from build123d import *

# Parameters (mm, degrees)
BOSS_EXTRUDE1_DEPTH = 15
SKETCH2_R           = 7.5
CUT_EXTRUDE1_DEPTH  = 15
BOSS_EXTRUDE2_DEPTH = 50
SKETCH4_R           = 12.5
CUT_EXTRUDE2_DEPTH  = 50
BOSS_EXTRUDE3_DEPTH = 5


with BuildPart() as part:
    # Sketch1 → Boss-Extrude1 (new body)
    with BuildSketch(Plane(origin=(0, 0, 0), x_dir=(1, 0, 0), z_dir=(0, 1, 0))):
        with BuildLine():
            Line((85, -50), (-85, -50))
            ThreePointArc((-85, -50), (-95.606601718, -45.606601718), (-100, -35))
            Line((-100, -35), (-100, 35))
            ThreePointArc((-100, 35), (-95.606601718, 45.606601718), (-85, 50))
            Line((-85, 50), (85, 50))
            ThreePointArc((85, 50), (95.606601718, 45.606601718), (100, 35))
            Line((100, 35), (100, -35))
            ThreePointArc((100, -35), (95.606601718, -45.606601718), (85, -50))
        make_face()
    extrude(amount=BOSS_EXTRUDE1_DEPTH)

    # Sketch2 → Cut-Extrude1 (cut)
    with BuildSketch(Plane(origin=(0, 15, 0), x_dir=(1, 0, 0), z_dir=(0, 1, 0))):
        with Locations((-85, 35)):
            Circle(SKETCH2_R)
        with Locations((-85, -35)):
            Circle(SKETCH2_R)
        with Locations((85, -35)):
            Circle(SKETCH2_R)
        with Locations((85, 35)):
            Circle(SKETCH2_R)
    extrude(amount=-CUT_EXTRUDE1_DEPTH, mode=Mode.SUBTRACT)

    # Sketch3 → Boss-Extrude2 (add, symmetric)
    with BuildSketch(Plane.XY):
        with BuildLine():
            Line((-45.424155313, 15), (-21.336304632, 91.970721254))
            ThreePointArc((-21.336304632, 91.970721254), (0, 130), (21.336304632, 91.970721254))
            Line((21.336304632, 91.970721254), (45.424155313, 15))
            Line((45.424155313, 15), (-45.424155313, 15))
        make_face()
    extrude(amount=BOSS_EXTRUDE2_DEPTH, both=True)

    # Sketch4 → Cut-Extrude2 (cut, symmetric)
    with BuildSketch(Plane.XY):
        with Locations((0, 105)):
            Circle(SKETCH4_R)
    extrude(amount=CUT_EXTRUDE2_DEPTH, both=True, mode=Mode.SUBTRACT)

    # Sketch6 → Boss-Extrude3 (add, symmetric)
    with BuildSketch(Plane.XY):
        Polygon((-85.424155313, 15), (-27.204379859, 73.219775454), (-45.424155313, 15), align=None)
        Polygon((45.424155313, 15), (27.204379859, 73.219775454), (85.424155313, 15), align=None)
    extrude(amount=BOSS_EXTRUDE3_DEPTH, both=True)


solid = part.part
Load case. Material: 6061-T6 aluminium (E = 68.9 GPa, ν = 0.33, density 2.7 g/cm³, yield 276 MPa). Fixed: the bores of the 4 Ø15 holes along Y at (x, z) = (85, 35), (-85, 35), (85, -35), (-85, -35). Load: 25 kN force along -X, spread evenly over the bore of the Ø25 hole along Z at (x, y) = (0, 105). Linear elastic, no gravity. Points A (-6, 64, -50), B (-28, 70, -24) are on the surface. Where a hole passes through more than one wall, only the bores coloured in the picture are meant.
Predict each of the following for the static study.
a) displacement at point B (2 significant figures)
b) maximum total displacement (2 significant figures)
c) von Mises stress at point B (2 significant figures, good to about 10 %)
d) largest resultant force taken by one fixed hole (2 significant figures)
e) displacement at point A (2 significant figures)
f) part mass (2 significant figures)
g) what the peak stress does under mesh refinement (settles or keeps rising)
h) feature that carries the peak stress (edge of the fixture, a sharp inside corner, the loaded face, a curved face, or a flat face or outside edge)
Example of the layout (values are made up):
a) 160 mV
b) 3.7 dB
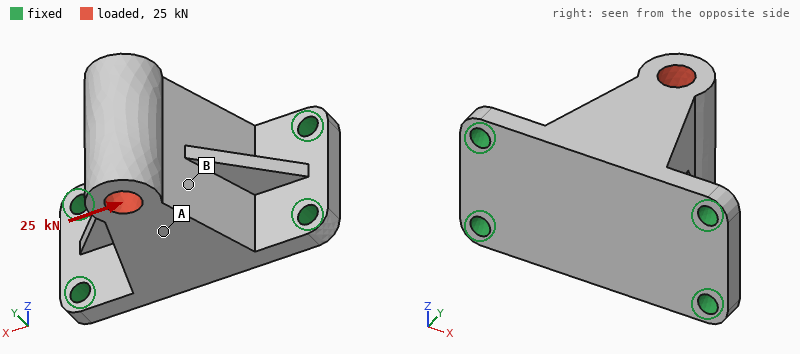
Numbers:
a) 0.082 mm
b) 0.18 mm
c) 18 MPa
d) 11 kN
e) 0.063 mm
f) 2.5 kg
g) keeps rising
h) edge of the fixture
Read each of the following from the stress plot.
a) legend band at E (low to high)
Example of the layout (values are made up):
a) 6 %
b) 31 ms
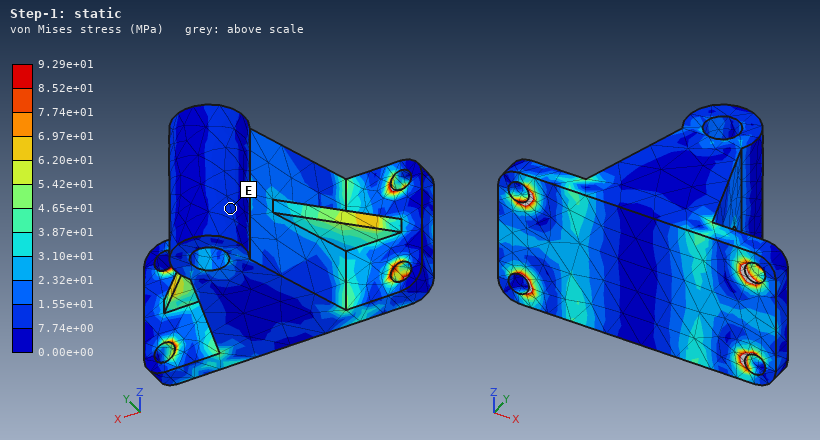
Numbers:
a) 7.74e+00 to 1.55e+01 MPa
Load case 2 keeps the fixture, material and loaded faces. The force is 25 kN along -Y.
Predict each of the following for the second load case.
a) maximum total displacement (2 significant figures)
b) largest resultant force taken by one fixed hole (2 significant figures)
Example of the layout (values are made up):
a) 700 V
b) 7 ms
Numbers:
a) 62 µm
b) 7.4 kN
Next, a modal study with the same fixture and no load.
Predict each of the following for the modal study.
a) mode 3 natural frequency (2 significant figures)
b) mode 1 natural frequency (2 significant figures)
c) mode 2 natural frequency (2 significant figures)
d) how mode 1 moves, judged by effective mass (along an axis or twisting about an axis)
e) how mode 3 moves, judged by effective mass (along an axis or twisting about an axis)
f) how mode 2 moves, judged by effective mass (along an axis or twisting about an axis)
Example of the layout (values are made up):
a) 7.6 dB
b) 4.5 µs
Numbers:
a) 2600 Hz
b) 1200 Hz
c) 2300 Hz
d) along Z
e) along X
f) along Y
